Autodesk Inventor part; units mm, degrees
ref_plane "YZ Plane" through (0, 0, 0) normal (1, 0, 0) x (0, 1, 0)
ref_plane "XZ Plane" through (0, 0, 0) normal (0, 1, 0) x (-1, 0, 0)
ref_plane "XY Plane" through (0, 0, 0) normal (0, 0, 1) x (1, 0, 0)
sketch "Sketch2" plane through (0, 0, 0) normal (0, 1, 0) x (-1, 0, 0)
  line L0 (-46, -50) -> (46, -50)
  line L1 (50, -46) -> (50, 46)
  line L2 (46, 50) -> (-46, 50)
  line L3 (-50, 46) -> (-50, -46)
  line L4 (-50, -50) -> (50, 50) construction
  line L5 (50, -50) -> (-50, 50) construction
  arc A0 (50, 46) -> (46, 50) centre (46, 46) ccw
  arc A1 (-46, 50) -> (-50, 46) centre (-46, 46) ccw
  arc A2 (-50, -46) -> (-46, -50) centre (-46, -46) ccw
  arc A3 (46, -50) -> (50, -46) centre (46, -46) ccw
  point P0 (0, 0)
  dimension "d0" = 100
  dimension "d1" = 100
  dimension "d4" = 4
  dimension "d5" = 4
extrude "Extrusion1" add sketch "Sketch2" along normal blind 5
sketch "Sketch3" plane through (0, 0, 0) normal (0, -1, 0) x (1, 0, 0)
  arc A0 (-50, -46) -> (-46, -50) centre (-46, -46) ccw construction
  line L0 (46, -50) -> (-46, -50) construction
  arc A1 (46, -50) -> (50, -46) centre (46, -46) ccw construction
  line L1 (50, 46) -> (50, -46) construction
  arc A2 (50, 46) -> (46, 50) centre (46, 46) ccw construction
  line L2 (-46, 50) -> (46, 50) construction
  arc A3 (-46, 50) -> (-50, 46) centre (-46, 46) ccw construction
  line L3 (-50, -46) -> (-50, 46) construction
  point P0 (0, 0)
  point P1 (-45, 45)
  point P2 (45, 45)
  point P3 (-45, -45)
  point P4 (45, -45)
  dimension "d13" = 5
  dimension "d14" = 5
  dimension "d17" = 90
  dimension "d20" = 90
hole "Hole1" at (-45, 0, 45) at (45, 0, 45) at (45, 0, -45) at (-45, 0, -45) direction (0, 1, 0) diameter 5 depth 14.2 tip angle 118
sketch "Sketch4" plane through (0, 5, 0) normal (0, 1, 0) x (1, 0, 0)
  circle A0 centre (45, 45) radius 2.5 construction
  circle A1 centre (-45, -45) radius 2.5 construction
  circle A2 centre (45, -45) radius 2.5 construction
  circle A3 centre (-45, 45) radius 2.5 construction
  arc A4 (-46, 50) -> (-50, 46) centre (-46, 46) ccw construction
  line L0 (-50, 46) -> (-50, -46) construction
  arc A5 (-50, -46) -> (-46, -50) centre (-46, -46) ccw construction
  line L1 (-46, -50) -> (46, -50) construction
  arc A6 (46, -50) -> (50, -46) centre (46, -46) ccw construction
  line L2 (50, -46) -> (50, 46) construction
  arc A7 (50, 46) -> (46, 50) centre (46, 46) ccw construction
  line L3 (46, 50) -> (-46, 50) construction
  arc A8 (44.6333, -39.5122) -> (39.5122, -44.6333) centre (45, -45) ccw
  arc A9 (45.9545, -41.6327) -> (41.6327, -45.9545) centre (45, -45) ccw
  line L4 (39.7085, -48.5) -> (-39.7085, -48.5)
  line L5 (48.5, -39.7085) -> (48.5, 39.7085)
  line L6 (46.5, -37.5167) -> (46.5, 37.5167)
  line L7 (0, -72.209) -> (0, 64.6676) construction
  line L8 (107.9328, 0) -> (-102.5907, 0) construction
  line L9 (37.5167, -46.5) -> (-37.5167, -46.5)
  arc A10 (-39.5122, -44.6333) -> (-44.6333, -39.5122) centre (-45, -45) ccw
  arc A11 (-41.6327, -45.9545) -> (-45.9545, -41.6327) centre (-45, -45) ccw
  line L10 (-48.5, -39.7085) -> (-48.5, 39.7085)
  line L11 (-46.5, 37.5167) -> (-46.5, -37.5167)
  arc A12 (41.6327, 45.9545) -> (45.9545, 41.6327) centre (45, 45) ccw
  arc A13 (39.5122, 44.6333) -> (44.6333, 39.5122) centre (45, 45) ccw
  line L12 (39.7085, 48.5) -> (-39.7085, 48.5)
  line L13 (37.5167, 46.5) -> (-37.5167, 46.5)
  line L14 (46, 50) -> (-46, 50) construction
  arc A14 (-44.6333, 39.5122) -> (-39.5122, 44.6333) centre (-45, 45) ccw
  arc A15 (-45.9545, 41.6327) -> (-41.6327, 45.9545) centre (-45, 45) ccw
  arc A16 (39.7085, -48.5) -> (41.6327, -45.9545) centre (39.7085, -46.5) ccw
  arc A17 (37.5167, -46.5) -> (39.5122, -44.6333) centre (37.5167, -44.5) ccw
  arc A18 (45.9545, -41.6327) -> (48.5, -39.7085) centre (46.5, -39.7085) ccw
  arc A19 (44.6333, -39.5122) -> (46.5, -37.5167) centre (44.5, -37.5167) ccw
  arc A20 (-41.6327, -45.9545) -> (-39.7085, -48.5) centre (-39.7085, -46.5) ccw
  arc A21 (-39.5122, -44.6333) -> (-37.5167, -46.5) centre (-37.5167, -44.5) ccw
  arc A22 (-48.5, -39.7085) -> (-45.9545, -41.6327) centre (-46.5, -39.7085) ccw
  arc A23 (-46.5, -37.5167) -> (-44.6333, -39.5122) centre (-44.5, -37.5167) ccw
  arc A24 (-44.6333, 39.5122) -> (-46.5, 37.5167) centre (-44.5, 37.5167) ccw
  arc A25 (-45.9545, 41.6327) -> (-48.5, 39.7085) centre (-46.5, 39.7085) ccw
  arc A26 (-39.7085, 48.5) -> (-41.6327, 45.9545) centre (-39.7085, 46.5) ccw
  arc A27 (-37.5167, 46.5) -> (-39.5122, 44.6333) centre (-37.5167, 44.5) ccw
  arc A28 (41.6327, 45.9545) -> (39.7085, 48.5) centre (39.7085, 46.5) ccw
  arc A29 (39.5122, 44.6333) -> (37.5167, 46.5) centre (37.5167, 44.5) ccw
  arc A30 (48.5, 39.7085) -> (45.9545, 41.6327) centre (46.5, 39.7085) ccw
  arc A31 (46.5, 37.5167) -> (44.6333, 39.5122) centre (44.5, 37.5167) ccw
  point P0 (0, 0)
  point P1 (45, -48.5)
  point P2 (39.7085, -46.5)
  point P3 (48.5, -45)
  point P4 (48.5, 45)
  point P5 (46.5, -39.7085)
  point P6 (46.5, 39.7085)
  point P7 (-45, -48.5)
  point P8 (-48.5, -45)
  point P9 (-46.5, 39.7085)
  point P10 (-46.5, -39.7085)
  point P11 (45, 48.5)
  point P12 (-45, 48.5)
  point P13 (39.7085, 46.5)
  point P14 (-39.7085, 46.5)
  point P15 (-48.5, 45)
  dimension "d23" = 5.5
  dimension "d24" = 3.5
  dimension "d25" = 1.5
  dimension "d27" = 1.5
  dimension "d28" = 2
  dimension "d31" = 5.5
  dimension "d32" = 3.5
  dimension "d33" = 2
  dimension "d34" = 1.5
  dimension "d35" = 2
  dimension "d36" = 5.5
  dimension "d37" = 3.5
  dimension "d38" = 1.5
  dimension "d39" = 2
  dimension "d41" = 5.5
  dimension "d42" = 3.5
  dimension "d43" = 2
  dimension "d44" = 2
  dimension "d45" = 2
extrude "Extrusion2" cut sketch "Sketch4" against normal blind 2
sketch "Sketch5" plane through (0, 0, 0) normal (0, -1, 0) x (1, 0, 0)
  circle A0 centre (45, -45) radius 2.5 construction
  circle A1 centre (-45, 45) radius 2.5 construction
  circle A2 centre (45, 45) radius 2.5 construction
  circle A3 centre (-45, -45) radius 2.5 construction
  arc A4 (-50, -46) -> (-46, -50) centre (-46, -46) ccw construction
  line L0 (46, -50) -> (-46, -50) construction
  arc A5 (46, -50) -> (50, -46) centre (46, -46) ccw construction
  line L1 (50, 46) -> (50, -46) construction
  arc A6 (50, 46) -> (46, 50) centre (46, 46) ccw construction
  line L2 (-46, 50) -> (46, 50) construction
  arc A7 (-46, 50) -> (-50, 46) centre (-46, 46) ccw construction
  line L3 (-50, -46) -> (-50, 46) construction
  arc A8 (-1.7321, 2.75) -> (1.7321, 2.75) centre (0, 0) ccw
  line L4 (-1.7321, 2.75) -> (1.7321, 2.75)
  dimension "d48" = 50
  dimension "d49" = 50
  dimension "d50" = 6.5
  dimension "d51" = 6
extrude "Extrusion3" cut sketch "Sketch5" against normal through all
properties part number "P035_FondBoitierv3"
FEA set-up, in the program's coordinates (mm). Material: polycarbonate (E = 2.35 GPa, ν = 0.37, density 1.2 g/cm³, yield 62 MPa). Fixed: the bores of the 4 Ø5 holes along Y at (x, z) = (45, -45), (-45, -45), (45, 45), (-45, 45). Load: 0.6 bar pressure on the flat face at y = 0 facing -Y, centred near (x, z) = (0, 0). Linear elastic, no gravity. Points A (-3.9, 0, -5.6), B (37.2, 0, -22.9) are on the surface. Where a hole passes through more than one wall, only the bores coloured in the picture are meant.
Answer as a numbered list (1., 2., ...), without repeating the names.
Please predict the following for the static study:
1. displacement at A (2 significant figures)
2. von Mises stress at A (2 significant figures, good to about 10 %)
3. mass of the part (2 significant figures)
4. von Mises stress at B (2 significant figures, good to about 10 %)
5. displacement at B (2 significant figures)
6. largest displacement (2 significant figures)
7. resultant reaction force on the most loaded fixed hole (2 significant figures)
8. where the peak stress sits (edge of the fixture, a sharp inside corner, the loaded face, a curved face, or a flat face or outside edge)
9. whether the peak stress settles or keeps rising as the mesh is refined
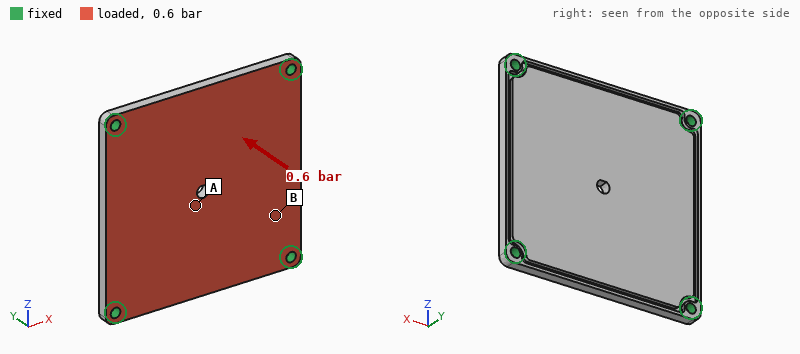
1. 1.6 mm
2. 8.1 MPa
3. 57 g
4. 3.8 MPa
5. 0.77 mm
6. 1.6 mm
7. 250 N
8. edge of the fixture
9. keeps rising
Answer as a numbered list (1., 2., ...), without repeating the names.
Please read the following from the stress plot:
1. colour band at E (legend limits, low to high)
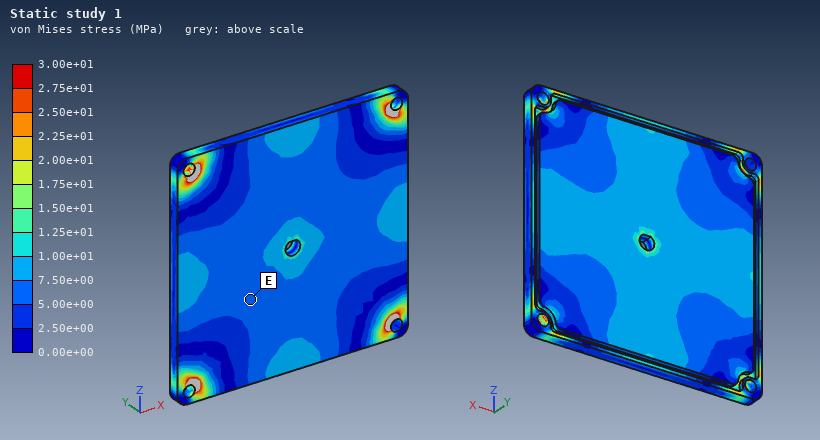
1. 5.00e+00 to 7.50e+00 MPa
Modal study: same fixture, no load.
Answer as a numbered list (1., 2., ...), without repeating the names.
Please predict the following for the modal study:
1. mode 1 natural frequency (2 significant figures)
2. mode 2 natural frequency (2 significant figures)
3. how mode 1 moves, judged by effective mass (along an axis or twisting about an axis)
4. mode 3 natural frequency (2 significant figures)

1. 480 Hz
2. 870 Hz
3. along Y
4. 870 Hz
